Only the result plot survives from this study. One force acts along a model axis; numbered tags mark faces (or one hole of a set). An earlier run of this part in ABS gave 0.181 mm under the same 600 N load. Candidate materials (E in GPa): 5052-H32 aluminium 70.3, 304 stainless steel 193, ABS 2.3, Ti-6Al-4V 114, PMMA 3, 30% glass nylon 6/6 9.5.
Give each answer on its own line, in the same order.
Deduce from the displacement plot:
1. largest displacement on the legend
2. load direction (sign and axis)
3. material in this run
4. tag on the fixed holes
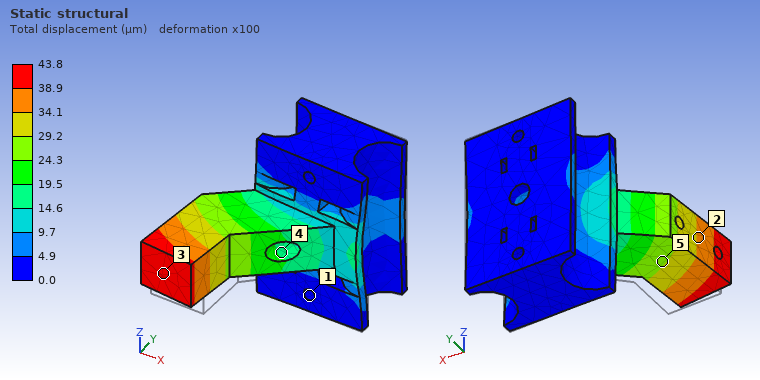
43.8 µm
-X
30% glass nylon 6/6
1
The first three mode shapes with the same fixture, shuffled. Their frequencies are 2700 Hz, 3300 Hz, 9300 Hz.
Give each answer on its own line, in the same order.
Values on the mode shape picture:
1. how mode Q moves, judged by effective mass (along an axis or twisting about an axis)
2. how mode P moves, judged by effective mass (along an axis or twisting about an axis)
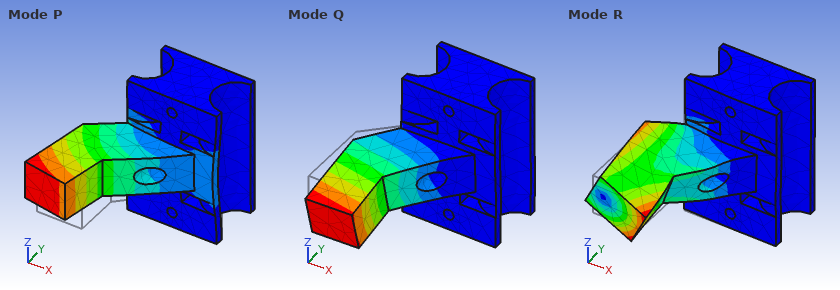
along Z
along X
